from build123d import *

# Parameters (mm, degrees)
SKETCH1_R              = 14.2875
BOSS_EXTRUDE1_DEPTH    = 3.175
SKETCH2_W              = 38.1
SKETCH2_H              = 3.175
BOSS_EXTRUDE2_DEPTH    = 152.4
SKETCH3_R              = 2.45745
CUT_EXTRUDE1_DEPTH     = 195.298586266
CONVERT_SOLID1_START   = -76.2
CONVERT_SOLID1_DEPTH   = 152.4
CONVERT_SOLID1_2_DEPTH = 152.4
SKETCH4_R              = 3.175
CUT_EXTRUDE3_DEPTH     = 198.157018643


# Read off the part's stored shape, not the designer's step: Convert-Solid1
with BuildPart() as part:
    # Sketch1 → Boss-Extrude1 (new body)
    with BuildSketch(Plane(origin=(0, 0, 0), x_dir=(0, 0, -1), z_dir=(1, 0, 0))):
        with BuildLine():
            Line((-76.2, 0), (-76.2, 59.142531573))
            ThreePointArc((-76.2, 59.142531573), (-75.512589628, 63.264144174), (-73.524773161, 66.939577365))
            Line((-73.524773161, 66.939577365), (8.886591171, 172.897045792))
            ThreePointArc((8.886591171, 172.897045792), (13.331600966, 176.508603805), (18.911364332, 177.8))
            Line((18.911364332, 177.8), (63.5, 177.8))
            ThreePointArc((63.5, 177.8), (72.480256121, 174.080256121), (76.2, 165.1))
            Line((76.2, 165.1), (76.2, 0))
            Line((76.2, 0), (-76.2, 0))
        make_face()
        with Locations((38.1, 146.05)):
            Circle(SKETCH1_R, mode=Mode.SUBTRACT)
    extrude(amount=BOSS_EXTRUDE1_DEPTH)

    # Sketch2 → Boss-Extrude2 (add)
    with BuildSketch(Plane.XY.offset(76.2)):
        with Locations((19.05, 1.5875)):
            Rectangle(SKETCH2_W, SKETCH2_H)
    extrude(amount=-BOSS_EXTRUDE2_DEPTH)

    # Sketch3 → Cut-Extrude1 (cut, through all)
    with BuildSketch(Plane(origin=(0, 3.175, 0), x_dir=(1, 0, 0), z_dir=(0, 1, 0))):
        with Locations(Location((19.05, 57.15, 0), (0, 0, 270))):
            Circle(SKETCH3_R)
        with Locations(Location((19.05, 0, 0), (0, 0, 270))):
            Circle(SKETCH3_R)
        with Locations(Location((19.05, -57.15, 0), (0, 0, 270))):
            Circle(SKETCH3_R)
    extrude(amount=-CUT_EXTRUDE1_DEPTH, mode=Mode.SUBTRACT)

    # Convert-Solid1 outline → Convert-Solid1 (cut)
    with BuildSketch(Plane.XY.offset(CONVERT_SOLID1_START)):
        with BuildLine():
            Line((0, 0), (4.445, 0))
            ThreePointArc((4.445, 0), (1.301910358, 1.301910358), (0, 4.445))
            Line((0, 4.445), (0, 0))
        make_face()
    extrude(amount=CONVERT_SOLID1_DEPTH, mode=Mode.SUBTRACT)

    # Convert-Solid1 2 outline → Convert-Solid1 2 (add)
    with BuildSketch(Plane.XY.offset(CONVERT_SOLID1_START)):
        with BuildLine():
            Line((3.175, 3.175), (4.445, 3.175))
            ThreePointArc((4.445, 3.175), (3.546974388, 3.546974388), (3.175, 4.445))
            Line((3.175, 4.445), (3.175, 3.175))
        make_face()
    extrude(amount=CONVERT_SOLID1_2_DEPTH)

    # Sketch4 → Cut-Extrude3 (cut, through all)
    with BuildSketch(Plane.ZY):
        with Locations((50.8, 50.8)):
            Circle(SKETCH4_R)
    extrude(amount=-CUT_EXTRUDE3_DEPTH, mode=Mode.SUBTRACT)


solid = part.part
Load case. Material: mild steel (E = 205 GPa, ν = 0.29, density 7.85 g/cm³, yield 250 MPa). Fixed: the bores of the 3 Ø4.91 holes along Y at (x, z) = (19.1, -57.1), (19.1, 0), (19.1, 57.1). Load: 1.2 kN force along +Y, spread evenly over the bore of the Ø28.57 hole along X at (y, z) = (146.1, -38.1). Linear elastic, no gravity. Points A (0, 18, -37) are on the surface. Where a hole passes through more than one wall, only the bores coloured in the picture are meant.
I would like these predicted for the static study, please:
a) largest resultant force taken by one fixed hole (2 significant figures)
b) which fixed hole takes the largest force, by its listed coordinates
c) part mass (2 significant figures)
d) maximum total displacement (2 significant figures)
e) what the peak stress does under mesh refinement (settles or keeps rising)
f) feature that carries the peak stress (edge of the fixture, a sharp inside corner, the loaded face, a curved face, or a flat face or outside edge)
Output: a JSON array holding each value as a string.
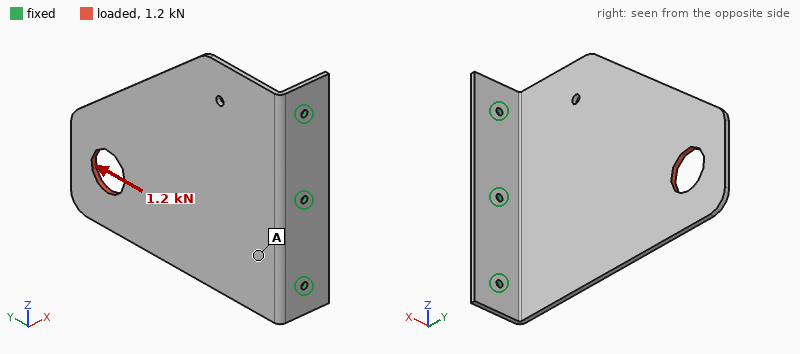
["790 N", "(19.1, -57.1)", "660 g", "0.59 mm", "keeps rising", "edge of the fixture"]
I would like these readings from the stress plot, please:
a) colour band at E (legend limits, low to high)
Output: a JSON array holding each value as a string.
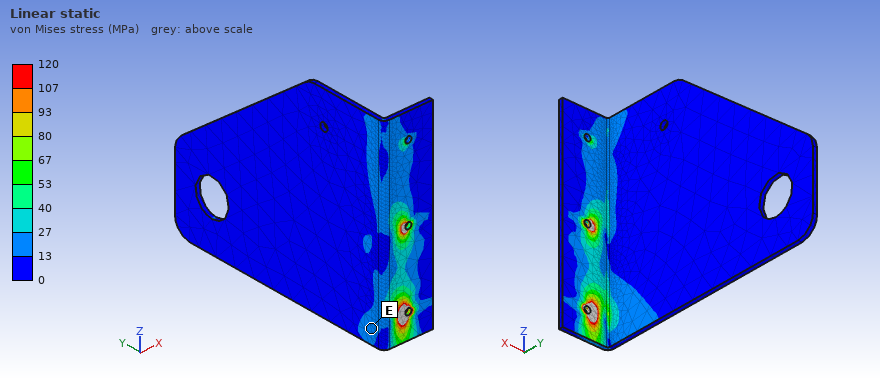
["13 to 27 MPa"]
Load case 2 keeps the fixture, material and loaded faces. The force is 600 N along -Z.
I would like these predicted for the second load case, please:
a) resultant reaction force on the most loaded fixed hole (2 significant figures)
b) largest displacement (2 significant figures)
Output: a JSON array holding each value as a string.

["770 N", "0.25 mm"]
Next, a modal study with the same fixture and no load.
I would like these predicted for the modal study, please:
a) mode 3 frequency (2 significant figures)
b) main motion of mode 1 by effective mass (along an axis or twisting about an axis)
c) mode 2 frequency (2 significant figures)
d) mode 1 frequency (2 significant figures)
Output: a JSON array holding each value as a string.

["510 Hz", "along X", "330 Hz", "95 Hz"]
